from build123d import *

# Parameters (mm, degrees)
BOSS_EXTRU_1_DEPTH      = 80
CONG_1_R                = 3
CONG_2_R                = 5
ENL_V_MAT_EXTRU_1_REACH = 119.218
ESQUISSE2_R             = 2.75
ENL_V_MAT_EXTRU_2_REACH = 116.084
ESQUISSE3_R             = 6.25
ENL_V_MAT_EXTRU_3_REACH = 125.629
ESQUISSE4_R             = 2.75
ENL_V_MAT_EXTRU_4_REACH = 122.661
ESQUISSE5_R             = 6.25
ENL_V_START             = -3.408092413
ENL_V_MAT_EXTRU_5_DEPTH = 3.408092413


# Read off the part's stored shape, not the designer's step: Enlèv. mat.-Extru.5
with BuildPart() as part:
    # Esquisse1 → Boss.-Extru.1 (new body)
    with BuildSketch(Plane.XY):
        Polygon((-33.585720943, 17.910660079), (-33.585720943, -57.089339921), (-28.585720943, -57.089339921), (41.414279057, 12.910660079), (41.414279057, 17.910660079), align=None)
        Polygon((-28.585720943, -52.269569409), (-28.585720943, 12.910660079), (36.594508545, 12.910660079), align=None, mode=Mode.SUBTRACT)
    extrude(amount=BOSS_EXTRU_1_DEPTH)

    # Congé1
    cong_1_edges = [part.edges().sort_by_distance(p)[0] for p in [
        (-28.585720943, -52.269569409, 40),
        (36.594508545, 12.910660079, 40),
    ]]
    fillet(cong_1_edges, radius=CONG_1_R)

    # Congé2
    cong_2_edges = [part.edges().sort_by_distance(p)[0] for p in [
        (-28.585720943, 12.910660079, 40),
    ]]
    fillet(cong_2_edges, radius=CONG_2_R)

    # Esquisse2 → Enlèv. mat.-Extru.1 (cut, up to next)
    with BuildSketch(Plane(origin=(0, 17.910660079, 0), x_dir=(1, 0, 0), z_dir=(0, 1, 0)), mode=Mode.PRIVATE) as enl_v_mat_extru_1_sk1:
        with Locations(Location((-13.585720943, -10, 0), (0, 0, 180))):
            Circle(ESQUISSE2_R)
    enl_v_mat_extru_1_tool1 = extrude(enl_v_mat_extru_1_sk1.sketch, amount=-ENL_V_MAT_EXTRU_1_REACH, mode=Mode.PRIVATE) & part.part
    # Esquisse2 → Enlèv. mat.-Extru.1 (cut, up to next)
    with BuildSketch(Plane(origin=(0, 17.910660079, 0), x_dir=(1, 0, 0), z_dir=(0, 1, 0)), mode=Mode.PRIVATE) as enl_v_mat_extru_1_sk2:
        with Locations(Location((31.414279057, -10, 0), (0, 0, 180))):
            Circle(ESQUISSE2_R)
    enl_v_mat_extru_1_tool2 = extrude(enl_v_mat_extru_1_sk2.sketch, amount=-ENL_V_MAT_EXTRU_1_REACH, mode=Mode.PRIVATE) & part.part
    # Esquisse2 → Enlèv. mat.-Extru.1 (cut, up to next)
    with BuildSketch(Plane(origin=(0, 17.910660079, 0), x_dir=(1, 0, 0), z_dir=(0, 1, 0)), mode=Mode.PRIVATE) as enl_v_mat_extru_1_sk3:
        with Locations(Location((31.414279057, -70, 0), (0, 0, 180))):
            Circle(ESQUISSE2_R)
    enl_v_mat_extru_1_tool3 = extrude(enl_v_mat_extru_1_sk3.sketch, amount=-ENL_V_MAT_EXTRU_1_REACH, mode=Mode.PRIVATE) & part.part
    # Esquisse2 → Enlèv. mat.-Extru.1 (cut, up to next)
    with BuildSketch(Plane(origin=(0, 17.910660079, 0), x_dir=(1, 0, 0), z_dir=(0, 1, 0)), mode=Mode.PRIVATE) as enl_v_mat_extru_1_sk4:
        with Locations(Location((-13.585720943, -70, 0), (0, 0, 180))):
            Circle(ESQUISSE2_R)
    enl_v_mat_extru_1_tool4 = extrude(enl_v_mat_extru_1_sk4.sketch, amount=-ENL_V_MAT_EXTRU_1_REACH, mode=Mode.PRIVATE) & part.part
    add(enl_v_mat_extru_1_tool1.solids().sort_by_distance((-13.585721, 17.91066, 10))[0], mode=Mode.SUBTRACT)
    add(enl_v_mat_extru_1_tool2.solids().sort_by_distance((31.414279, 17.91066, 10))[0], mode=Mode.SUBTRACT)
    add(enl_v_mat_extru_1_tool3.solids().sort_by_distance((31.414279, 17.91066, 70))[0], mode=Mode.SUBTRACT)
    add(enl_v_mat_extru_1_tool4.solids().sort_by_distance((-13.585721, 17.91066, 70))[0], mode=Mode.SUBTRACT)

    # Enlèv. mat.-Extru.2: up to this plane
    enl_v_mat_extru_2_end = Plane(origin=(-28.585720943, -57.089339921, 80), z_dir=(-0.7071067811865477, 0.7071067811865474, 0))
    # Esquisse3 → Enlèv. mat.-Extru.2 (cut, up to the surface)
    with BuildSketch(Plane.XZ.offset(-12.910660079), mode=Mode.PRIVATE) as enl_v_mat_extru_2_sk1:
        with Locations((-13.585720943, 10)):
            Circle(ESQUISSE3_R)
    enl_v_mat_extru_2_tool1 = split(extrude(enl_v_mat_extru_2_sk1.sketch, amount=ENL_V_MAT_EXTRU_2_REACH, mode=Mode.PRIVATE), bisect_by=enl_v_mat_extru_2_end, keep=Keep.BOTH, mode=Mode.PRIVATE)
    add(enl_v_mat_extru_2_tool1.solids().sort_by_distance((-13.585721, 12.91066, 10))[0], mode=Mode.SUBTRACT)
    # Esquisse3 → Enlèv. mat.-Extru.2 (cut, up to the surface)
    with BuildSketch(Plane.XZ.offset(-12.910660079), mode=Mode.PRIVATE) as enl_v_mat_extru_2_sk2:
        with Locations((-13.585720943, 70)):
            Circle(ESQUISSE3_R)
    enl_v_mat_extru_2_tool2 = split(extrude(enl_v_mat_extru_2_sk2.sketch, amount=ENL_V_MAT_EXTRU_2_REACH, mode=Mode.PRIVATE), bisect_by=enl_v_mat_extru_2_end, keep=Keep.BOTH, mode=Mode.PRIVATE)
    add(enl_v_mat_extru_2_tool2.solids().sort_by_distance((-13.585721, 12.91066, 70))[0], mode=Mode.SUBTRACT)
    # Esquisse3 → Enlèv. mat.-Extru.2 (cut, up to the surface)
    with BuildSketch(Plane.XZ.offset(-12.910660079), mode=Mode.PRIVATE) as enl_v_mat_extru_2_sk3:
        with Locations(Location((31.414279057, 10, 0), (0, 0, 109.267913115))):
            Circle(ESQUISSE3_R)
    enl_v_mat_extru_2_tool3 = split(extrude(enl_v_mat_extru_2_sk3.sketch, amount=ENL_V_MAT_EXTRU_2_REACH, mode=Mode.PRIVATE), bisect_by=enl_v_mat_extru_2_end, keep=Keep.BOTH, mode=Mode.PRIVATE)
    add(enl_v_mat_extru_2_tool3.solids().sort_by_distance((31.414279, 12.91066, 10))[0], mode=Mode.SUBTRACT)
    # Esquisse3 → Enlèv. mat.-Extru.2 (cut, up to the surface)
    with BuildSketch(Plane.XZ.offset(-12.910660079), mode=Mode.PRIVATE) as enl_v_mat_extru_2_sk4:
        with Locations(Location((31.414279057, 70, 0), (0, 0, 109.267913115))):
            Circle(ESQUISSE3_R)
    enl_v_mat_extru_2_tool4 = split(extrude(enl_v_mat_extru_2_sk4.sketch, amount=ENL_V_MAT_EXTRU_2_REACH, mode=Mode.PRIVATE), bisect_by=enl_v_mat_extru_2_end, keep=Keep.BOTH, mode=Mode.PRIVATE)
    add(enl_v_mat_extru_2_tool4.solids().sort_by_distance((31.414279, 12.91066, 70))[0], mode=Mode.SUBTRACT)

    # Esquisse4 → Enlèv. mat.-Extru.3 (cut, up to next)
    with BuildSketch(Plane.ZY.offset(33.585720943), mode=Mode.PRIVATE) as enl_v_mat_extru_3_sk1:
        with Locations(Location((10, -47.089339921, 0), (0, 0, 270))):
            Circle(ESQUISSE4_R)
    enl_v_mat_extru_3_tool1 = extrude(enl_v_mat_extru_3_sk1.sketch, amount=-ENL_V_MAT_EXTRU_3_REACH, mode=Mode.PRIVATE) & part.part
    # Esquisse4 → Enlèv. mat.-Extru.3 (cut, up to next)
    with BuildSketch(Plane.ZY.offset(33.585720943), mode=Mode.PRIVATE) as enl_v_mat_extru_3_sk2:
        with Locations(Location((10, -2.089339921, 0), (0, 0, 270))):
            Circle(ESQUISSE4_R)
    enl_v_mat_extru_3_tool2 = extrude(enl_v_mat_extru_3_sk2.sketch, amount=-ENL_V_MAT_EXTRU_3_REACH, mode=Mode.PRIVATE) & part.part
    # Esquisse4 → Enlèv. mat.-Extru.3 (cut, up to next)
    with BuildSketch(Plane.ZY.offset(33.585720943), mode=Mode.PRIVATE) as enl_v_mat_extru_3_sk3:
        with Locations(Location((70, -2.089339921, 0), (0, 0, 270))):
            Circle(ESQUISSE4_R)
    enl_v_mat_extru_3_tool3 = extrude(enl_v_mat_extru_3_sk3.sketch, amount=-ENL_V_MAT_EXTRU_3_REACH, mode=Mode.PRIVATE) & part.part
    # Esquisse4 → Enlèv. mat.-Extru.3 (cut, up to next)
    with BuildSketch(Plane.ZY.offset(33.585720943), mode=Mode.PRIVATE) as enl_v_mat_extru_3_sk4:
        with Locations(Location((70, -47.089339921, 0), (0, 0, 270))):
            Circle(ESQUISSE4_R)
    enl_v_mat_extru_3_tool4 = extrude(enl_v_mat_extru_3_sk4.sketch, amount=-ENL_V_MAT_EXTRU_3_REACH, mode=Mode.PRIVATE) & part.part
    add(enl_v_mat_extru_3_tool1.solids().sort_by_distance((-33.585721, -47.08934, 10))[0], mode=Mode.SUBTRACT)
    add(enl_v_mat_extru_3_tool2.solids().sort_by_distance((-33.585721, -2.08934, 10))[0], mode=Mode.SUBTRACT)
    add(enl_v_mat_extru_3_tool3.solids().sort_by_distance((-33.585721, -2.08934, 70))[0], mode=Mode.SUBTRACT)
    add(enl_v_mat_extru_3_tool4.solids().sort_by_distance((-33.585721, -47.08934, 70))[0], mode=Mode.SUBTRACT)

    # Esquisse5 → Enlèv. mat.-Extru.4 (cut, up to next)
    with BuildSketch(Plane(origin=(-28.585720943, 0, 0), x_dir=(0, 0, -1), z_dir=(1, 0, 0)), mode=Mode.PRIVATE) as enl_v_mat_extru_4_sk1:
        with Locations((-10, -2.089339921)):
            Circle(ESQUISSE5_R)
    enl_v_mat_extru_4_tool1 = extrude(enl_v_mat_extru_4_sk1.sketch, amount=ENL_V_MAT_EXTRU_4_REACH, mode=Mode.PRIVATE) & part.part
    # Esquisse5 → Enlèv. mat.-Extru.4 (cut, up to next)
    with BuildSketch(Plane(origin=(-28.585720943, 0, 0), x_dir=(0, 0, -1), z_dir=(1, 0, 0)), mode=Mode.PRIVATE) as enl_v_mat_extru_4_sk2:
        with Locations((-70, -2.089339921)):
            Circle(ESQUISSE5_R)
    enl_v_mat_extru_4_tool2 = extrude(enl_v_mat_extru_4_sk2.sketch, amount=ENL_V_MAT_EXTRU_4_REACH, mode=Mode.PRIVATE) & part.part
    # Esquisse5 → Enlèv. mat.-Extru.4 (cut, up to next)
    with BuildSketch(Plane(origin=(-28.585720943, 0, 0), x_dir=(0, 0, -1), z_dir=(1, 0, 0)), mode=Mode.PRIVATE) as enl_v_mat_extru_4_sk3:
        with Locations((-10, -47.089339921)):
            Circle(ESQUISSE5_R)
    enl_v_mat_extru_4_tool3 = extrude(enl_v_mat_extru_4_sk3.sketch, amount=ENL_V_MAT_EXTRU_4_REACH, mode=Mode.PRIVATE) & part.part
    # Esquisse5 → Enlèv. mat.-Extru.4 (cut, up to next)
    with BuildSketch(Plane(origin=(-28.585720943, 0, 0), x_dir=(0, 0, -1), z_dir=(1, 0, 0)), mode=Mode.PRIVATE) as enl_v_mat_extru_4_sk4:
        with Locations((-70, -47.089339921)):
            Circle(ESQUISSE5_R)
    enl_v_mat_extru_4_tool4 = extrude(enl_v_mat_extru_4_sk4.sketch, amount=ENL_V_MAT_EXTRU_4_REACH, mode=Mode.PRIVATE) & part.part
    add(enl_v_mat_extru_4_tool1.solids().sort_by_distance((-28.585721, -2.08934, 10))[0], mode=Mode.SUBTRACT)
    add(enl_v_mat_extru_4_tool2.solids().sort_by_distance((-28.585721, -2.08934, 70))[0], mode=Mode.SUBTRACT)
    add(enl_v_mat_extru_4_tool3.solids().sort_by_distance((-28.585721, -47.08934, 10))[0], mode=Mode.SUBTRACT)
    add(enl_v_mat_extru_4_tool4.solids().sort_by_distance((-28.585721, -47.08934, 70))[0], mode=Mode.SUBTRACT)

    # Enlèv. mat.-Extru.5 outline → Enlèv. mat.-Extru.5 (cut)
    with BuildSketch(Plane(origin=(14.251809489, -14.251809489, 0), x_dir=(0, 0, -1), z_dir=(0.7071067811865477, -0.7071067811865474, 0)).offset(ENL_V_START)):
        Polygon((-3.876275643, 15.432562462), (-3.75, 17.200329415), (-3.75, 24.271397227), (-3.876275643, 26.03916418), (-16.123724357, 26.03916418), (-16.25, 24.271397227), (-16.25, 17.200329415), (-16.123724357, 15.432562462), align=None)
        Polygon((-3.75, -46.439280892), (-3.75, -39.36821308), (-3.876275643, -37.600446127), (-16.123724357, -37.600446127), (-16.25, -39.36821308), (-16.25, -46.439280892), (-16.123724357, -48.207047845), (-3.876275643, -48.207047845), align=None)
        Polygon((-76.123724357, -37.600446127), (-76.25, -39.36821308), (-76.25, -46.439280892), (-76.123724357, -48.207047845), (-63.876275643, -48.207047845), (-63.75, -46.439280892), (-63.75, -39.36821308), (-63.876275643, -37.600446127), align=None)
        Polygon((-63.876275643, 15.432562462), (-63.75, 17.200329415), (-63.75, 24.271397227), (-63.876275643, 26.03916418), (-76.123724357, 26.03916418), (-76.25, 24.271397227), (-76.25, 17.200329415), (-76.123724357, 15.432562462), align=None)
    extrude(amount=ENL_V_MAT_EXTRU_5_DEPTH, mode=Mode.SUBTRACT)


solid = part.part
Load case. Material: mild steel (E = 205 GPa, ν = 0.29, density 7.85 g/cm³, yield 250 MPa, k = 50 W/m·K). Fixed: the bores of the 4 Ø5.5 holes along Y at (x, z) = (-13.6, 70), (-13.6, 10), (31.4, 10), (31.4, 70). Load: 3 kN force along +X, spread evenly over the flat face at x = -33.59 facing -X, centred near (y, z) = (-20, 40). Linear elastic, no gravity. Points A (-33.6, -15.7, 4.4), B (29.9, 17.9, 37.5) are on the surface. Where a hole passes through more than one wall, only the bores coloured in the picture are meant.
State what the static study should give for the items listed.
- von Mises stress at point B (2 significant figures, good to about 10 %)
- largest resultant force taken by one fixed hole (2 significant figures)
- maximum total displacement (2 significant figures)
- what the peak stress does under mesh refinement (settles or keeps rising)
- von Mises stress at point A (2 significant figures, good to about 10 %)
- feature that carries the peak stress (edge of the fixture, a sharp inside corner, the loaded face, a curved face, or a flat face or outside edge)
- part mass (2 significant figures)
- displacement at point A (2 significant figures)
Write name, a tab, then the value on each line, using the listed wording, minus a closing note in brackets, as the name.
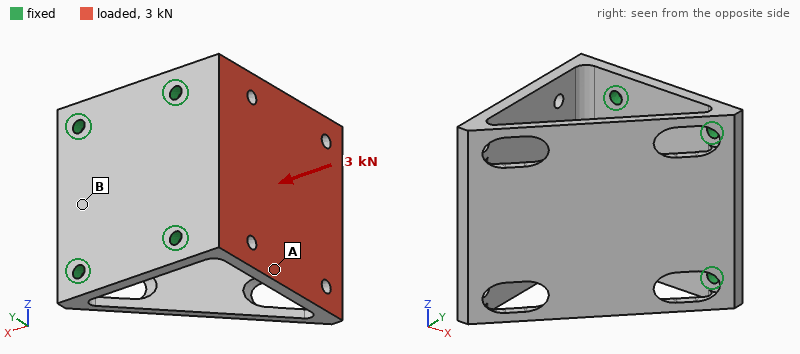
von Mises stress at point B	17 MPa
largest resultant force taken by one fixed hole	1.1 kN
maximum total displacement	83 µm
what the peak stress does under mesh refinement	keeps rising
von Mises stress at point A	45 MPa
feature that carries the peak stress	edge of the fixture
part mass	630 g
displacement at point A	76 µm
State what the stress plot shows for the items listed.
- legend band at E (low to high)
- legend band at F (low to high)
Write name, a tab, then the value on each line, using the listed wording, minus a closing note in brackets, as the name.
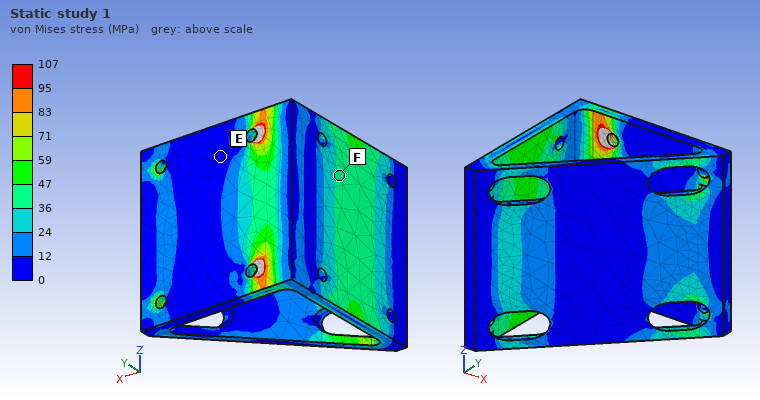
legend band at E	0 to 12 MPa
legend band at F	36 to 47 MPa
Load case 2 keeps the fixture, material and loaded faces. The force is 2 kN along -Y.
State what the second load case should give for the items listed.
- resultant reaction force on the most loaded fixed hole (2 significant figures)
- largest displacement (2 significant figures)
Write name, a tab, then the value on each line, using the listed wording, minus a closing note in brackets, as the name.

resultant reaction force on the most loaded fixed hole	1.2 kN
largest displacement	37 µm
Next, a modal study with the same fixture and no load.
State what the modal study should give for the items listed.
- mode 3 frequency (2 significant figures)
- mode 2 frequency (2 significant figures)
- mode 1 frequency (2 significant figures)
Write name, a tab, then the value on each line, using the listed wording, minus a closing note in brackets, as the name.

mode 3 frequency	2500 Hz
mode 2 frequency	2400 Hz
mode 1 frequency	1500 Hz
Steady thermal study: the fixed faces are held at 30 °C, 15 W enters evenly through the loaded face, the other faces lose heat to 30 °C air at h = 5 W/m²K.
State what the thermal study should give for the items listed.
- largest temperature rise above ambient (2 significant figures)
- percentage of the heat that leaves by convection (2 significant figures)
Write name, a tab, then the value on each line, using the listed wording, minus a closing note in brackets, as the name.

largest temperature rise above ambient	26 K
percentage of the heat that leaves by convection	12 %
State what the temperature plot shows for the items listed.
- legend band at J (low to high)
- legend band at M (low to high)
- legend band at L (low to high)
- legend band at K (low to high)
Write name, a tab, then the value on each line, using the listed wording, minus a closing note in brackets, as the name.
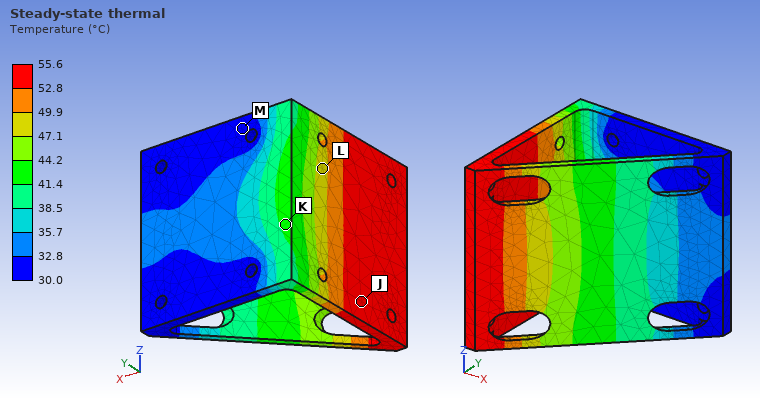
legend band at J	52.8 to 55.6 °C
legend band at M	30.0 to 32.8 °C
legend band at L	47.1 to 49.9 °C
legend band at K	41.4 to 44.2 °C
